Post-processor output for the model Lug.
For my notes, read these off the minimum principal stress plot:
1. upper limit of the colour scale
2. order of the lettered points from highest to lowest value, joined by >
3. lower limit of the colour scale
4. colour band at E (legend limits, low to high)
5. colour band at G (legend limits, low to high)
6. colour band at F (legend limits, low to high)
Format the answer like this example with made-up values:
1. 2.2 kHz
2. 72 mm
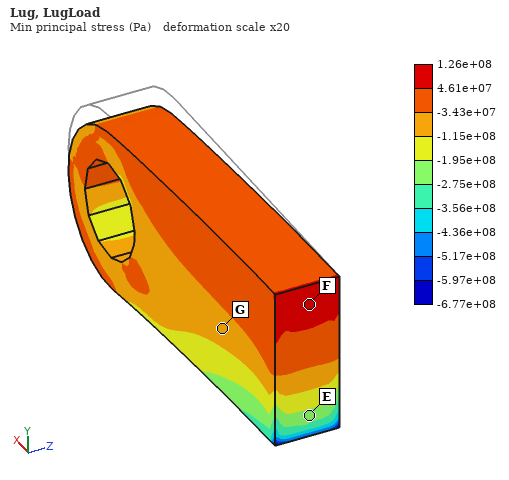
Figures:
1. 1.26e+08 Pa
2. F > G > E
3. -6.77e+08 Pa
4. -2.75e+08 to -1.95e+08 Pa
5. -1.15e+08 to -3.43e+07 Pa
6. 4.61e+07 to 1.26e+08 Pa
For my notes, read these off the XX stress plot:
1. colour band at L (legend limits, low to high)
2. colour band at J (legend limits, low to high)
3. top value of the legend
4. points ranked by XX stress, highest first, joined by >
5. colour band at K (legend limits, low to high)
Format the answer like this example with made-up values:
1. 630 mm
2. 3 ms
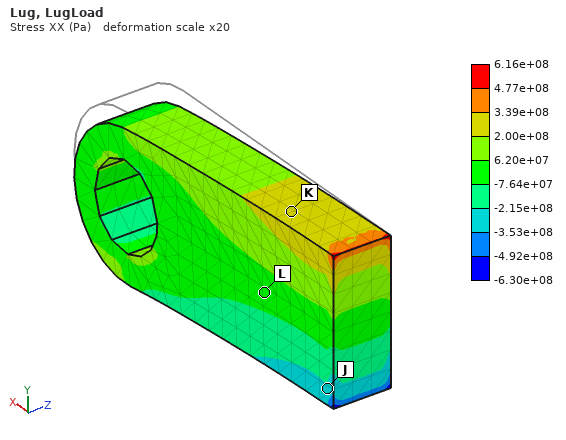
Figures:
1. -7.64e+07 to 6.20e+07 Pa
2. -3.53e+08 to -2.15e+08 Pa
3. 6.16e+08 Pa
4. K > L > J
5. 2.00e+08 to 3.39e+08 Pa
